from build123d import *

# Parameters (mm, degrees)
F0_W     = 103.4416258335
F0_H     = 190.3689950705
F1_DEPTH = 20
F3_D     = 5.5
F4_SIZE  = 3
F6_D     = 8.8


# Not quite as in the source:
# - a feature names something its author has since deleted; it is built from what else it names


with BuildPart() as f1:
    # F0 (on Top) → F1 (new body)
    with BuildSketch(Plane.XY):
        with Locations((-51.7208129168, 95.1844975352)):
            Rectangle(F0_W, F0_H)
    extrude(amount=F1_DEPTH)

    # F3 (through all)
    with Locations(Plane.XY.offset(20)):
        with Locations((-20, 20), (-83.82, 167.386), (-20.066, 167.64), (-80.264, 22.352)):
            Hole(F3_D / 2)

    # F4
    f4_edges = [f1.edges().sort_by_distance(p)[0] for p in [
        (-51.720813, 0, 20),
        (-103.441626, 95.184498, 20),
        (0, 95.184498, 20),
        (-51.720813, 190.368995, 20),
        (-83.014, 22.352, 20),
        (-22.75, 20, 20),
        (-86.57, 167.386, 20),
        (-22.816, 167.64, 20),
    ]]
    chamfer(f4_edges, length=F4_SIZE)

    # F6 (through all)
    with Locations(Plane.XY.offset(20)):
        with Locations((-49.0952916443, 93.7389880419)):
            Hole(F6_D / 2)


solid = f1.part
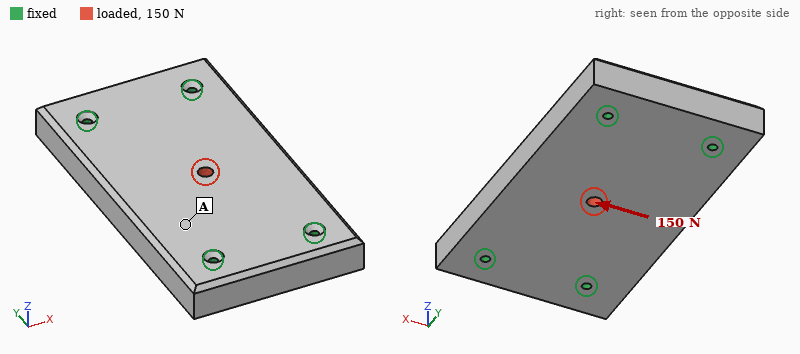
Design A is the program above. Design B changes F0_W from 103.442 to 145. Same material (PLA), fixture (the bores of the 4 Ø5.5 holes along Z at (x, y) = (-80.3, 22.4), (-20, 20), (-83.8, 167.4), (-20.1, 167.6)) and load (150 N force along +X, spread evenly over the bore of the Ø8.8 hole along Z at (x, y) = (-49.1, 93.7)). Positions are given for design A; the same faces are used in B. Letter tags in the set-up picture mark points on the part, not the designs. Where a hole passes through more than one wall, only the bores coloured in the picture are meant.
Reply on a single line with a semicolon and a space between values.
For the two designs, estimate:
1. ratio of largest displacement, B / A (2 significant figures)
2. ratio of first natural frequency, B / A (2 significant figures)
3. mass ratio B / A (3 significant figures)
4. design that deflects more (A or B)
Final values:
0.80; 0.88; 1.41; A
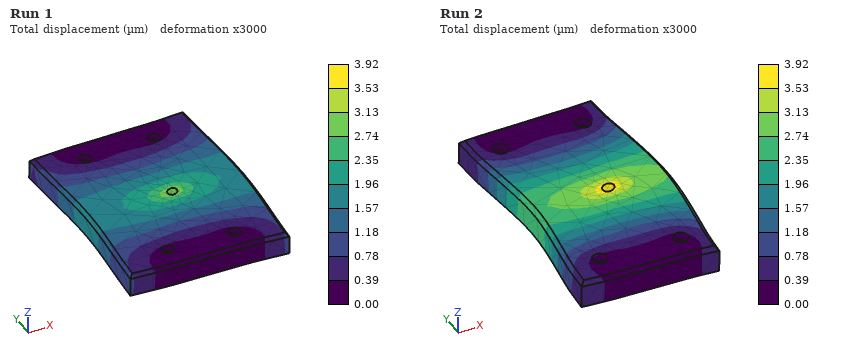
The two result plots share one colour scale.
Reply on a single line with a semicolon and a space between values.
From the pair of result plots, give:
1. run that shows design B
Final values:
Run 1
